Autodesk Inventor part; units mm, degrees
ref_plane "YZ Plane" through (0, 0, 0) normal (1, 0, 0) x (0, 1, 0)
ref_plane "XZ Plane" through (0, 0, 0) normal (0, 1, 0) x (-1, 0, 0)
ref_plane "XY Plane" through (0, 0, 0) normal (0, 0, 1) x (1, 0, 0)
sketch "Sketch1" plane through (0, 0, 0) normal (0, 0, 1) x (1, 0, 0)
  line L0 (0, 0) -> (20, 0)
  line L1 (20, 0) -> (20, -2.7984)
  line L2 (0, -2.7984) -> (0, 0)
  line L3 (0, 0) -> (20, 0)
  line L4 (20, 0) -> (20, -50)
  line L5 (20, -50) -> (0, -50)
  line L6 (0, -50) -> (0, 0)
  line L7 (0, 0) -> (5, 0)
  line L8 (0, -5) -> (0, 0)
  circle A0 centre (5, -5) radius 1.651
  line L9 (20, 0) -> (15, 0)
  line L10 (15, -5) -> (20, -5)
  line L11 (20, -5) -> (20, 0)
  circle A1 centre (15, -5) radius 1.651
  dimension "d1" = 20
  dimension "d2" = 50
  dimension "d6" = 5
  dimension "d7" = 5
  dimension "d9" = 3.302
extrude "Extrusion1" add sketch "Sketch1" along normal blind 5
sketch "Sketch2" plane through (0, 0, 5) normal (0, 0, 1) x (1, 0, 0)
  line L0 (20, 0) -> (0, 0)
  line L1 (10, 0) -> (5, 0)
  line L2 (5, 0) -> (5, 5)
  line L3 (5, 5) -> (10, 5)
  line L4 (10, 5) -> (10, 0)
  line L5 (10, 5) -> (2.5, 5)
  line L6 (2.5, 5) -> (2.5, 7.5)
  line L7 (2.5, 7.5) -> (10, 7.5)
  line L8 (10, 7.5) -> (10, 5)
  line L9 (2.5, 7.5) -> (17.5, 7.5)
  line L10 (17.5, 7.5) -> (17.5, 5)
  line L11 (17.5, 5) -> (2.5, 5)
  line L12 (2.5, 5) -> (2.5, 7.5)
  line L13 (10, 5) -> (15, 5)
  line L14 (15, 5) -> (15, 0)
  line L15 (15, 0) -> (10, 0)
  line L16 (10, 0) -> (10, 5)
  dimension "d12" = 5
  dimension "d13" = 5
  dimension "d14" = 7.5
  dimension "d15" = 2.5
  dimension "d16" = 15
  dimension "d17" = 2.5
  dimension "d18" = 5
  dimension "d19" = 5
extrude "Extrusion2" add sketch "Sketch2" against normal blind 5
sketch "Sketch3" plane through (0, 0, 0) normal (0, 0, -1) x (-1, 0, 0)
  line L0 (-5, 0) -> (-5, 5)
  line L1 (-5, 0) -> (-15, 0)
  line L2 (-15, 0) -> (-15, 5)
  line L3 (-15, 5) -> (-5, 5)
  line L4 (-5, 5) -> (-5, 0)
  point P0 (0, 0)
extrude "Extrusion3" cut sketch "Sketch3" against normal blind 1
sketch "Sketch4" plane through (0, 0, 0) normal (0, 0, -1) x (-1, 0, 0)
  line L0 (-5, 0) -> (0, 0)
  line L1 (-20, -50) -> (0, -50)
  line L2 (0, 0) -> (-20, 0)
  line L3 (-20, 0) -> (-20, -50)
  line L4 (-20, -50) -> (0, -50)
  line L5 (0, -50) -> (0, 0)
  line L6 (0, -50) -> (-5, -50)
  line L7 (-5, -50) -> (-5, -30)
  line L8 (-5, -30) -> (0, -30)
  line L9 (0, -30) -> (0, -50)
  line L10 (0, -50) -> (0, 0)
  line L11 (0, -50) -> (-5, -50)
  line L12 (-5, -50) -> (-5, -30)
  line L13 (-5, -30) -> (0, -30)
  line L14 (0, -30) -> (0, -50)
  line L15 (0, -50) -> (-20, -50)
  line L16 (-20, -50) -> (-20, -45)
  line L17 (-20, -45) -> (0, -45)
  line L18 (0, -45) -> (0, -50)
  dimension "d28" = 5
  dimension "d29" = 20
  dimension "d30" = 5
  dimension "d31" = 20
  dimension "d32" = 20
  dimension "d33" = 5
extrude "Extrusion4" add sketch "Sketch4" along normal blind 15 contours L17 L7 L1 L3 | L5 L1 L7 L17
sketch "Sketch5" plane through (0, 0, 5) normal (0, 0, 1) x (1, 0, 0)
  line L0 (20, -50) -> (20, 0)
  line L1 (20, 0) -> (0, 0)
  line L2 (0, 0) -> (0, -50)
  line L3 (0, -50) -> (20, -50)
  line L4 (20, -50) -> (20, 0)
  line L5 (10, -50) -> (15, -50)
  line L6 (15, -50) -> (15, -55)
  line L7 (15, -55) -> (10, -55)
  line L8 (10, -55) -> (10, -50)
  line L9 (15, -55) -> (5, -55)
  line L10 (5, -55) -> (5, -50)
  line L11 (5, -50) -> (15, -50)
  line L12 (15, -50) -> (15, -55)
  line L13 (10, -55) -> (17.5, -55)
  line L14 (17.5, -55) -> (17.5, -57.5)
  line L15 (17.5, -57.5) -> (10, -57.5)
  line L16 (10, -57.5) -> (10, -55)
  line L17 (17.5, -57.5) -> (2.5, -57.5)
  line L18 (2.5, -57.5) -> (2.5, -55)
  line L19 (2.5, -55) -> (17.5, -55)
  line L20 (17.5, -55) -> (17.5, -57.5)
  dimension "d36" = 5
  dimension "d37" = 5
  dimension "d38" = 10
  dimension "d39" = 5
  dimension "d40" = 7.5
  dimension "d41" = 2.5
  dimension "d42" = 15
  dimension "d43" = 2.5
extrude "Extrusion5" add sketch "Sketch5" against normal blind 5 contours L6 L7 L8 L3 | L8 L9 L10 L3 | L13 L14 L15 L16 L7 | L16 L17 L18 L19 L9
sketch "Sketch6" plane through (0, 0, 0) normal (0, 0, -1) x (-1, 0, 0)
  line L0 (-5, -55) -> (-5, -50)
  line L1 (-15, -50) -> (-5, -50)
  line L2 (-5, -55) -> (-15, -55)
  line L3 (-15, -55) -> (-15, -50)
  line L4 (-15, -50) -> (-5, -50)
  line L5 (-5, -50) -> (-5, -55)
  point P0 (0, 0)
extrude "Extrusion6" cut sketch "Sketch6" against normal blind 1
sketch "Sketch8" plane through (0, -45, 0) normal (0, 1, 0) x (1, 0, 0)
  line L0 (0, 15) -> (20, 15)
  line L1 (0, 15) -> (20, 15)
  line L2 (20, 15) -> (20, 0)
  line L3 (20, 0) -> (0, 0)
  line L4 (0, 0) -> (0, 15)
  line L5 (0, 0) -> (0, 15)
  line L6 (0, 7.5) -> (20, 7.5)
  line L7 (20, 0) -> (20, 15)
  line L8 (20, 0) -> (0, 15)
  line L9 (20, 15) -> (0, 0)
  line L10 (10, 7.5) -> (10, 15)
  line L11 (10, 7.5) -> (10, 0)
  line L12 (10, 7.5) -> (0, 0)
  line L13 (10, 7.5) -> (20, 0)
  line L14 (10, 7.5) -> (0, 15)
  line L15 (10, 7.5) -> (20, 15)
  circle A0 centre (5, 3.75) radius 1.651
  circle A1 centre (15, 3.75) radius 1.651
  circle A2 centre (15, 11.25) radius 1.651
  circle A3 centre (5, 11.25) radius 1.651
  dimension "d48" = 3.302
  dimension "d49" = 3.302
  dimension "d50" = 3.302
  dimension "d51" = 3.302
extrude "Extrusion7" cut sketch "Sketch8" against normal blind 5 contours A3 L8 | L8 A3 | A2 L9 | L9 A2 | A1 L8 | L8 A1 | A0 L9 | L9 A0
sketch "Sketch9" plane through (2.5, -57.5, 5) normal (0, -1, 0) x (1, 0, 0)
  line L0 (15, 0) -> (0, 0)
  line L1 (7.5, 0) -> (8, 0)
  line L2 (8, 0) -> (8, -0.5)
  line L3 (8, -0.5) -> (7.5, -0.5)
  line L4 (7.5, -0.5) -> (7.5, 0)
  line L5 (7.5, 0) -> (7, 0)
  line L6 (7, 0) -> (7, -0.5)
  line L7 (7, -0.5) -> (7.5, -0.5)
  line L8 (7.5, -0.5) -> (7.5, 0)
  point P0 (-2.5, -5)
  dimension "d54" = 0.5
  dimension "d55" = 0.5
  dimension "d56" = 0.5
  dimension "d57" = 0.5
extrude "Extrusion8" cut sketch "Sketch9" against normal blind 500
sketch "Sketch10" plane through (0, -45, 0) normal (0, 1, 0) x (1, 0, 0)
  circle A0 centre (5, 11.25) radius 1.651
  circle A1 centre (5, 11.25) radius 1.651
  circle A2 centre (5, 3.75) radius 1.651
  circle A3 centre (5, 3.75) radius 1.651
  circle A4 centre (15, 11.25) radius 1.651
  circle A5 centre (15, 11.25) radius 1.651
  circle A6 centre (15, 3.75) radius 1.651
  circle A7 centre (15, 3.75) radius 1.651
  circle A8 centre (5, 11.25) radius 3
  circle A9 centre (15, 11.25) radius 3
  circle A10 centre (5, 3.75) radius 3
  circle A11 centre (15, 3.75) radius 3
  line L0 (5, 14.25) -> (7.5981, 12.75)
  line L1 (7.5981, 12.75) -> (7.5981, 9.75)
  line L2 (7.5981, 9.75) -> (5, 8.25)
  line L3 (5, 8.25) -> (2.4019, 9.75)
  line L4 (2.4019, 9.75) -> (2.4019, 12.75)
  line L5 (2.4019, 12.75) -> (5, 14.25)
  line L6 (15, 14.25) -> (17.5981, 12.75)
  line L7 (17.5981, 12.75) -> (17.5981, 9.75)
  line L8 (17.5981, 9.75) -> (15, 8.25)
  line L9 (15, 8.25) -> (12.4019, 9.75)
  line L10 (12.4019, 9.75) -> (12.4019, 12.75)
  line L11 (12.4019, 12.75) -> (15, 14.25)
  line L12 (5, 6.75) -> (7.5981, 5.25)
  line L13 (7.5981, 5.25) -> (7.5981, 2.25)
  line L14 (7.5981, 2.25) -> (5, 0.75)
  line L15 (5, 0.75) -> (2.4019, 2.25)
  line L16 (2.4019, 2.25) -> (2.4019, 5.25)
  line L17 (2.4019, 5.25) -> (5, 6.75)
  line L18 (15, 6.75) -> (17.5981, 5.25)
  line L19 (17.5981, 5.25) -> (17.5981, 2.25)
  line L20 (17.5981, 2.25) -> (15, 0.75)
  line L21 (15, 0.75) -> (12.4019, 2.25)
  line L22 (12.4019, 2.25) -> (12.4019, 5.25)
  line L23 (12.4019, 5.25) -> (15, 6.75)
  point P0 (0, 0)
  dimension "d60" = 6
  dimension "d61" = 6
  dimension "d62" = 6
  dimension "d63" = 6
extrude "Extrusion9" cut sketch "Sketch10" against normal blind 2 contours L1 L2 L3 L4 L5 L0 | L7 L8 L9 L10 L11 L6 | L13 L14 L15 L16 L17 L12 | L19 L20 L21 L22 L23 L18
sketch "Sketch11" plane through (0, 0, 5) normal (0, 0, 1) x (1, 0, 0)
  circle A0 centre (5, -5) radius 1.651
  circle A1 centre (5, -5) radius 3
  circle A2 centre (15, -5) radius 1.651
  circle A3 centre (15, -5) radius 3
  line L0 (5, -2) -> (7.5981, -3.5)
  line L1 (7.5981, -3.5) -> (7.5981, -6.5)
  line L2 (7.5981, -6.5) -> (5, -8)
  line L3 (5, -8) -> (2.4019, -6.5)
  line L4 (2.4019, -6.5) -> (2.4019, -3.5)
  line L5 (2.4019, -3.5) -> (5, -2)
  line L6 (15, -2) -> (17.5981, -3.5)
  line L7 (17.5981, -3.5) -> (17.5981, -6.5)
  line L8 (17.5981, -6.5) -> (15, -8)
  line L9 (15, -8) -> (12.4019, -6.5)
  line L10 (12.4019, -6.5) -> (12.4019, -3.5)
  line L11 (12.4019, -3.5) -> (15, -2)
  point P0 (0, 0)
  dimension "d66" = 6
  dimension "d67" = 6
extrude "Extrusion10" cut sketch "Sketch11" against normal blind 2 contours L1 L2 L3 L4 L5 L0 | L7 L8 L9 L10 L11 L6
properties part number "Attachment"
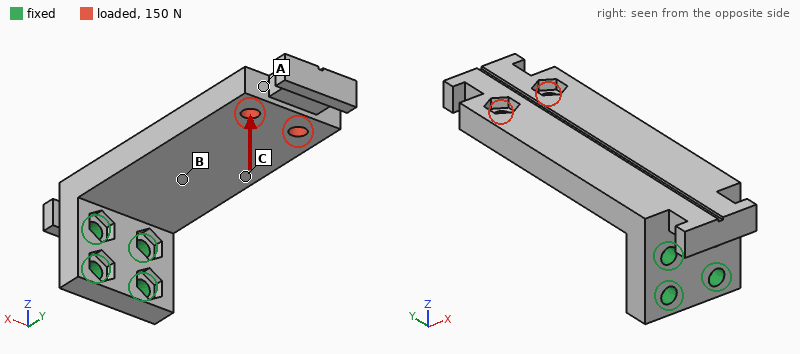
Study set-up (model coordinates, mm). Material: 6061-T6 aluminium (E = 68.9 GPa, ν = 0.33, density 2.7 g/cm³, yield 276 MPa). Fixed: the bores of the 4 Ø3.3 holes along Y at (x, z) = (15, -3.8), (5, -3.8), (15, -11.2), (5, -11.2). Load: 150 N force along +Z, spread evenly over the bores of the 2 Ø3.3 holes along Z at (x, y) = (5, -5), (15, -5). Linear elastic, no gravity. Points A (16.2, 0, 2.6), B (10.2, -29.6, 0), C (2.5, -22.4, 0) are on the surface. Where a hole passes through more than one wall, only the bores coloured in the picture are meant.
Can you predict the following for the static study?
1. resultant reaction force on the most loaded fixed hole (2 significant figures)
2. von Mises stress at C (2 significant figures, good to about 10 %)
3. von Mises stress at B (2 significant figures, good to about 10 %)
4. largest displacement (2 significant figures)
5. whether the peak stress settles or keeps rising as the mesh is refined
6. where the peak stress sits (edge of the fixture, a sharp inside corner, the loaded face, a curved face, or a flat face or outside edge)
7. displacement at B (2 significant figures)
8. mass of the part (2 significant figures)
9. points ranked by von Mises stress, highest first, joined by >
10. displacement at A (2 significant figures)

280 N
32 MPa
44 MPa
0.56 mm
keeps rising
edge of the fixture
0.12 mm
18 g
B > C > A
0.46 mm
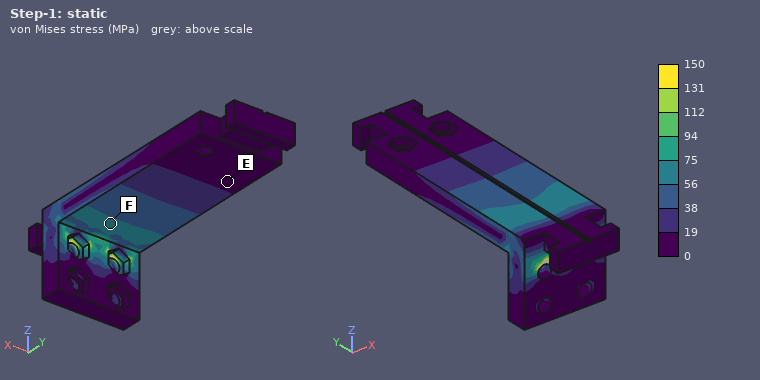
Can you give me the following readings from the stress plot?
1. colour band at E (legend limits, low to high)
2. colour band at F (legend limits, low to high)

0 to 19 MPa
56 to 75 MPa
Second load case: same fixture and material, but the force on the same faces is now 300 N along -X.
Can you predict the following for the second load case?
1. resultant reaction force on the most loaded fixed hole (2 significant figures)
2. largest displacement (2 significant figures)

1.1 kN
0.16 mm
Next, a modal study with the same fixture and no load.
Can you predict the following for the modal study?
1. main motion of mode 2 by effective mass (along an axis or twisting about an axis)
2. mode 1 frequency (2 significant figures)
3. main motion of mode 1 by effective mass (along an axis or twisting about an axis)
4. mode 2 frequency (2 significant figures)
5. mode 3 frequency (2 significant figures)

along X
1300 Hz
along Z
3200 Hz
7000 Hz
